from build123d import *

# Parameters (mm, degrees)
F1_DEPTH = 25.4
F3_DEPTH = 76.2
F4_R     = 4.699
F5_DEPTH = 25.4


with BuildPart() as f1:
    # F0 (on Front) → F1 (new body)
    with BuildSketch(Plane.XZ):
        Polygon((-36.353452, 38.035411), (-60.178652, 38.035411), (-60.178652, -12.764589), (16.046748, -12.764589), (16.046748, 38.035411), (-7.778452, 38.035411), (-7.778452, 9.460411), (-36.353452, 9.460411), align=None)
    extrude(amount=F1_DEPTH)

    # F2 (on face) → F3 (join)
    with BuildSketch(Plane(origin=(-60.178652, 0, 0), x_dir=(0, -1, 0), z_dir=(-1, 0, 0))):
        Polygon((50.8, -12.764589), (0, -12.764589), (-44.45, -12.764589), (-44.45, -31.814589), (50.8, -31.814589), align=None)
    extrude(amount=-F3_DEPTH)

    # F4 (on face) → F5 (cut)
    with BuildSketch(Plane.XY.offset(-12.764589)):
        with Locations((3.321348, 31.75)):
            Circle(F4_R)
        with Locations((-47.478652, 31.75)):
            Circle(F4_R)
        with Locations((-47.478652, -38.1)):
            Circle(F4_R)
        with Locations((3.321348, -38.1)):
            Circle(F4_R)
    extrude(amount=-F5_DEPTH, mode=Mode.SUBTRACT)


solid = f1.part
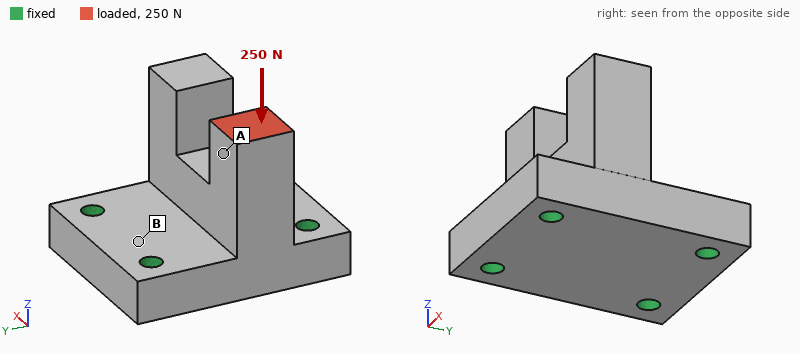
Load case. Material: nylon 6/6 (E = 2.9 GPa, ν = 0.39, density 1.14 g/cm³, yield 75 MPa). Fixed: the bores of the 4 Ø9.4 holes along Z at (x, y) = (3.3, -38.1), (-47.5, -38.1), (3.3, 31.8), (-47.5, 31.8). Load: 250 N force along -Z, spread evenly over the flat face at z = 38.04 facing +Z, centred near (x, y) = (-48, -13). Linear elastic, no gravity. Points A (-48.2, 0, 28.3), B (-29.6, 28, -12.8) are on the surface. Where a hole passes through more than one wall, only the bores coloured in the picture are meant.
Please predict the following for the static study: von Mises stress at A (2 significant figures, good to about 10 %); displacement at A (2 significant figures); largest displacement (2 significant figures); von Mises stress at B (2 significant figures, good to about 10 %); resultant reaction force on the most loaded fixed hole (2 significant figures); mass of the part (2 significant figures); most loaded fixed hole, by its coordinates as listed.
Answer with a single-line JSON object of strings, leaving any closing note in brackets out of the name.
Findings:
{"von Mises stress at A": "0.41 MPa", "displacement at A": "19 µm", "largest displacement": "25 µm", "von Mises stress at B": "0.10 MPa", "resultant reaction force on the most loaded fixed hole": "160 N", "mass of the part": "240 g", "most loaded fixed hole, by its coordinates as listed": "(-47.5, -38.1)"}
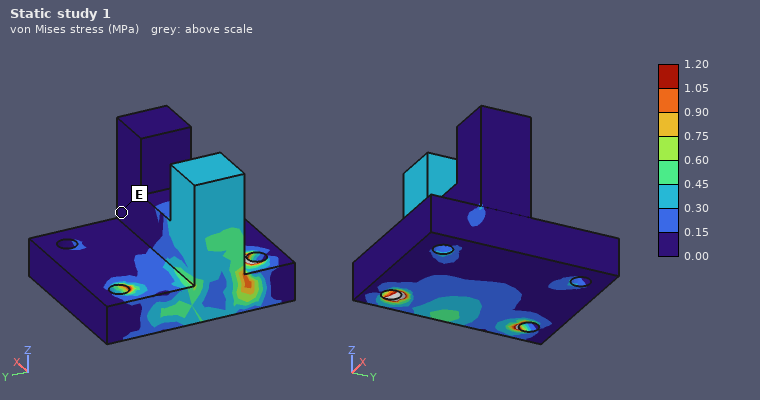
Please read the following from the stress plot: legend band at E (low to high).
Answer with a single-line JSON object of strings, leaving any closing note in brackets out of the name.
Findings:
{"legend band at E": "0.00 to 0.15 MPa"}
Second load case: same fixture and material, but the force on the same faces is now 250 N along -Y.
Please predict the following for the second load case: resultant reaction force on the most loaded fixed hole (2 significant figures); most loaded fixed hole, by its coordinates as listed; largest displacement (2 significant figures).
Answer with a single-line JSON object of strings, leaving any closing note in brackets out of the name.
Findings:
{"resultant reaction force on the most loaded fixed hole": "220 N", "most loaded fixed hole, by its coordinates as listed": "(-47.5, -38.1)", "largest displacement": "0.17 mm"}
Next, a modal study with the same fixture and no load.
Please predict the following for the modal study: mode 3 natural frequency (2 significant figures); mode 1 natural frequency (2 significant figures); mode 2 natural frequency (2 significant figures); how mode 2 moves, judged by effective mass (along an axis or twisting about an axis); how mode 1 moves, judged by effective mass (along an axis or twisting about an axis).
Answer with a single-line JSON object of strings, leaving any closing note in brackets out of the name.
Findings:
{"mode 3 natural frequency": "2100 Hz", "mode 1 natural frequency": "1800 Hz", "mode 2 natural frequency": "1900 Hz", "how mode 2 moves, judged by effective mass": "along X", "how mode 1 moves, judged by effective mass": "along Y"}
